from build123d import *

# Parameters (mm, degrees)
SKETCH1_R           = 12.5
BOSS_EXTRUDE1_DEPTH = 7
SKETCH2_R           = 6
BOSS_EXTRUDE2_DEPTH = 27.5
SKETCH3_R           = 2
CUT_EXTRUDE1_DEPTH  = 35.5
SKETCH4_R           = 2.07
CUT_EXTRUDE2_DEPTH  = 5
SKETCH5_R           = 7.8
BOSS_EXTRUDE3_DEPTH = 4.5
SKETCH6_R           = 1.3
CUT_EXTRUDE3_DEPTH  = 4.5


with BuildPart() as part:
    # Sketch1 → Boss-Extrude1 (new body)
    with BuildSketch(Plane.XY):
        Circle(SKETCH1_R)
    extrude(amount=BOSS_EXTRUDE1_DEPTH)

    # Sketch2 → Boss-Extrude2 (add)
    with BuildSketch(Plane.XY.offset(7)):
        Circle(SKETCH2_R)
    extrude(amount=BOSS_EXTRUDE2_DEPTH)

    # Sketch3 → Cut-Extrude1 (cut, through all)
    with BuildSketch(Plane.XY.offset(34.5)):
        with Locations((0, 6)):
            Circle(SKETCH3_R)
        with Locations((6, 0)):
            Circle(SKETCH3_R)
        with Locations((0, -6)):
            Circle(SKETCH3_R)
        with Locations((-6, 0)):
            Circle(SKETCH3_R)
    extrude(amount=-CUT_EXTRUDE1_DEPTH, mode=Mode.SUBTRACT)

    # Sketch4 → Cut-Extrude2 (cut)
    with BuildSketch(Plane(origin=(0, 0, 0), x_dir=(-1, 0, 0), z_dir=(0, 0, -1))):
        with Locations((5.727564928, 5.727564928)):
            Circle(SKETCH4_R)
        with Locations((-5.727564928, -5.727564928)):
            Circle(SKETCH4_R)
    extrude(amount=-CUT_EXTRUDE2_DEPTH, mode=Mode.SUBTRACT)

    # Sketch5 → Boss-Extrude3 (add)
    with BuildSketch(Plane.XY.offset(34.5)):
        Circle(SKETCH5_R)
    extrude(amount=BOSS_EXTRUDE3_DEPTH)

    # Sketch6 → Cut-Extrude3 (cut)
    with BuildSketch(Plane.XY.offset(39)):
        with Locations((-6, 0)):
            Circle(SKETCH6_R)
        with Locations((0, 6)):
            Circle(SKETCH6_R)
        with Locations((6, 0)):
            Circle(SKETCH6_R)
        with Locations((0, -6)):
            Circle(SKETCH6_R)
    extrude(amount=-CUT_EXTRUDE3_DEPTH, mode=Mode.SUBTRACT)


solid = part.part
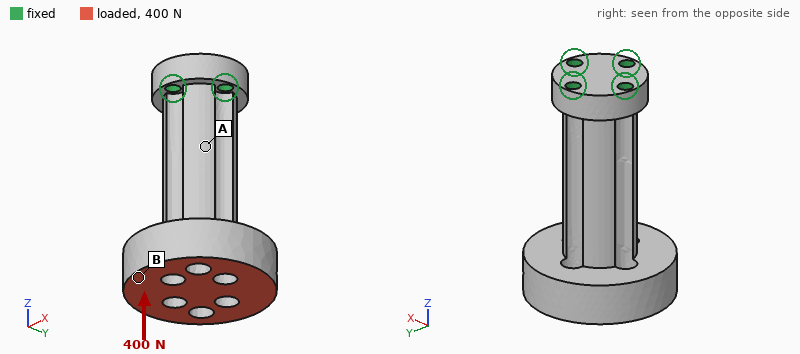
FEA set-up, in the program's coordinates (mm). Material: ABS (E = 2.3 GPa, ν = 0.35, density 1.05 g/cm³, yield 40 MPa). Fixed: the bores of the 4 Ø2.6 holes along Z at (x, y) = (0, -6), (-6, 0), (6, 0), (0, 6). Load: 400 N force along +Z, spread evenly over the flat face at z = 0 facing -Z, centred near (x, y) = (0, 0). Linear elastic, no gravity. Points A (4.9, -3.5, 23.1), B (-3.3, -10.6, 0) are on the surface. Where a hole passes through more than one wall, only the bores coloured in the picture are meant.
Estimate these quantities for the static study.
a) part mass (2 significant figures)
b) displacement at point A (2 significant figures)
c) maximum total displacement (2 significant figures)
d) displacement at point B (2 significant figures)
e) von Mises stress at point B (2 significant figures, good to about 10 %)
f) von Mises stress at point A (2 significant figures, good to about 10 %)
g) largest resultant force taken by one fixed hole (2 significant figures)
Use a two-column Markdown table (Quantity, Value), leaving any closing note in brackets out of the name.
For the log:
| Quantity | Value |
|---|---|
| part mass | 6.5 g |
| displacement at point A | 30 µm |
| maximum total displacement | 94 µm |
| displacement at point B | 90 µm |
| von Mises stress at point B | 2.1 MPa |
| von Mises stress at point A | 4.4 MPa |
| largest resultant force taken by one fixed hole | 110 N |
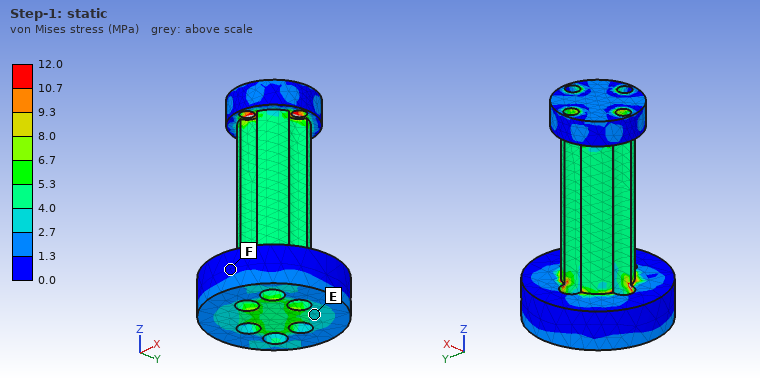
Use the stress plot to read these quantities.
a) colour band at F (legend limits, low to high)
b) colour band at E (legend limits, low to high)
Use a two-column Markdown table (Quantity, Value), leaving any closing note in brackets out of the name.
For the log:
| Quantity | Value |
|---|---|
| colour band at F | 0.0 to 1.3 MPa |
| colour band at E | 2.7 to 4.0 MPa |
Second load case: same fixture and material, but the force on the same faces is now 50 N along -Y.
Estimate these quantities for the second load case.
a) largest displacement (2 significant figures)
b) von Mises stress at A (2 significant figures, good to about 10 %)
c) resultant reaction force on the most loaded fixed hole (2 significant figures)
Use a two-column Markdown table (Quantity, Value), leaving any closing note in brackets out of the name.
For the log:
| Quantity | Value |
|---|---|
| largest displacement | 0.60 mm |
| von Mises stress at A | 5.7 MPa |
| resultant reaction force on the most loaded fixed hole | 140 N |
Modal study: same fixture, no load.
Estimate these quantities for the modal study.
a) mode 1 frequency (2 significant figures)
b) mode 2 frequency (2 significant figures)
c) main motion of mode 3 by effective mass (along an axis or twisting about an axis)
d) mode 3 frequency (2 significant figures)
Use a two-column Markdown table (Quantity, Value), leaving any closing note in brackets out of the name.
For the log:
| Quantity | Value |
|---|---|
| mode 1 frequency | 900 Hz |
| mode 2 frequency | 910 Hz |
| main motion of mode 3 by effective mass | twisting about Z |
| mode 3 frequency | 1600 Hz |
